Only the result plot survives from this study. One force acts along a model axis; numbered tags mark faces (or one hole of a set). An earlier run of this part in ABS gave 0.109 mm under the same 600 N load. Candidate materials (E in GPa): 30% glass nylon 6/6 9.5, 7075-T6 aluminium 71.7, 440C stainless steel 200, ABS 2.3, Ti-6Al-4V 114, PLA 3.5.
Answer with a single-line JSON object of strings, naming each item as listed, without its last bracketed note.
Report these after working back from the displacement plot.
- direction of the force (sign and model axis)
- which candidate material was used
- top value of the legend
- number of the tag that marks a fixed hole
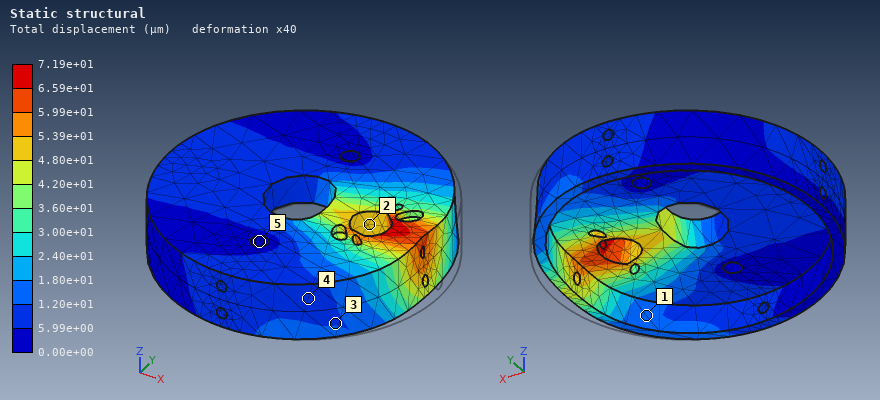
{"direction of the force": "-X", "which candidate material was used": "PLA", "top value of the legend": "7.19e+01 µm", "number of the tag that marks a fixed hole": "5"}
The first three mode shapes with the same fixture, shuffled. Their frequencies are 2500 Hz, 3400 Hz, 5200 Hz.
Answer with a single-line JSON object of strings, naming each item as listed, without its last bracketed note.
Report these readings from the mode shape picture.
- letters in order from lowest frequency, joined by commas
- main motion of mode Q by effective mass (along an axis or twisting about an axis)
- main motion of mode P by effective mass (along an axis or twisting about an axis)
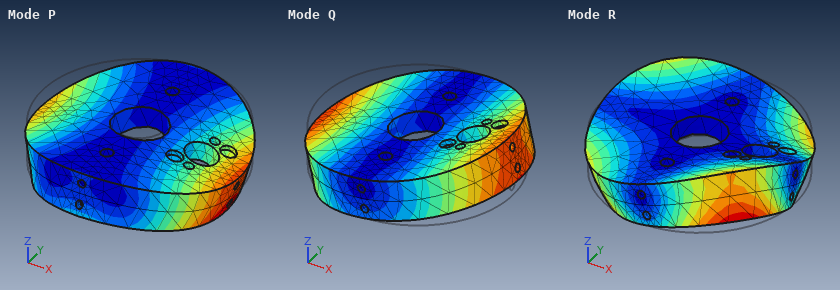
{"letters in order from lowest frequency, joined by commas": "Q, P, R", "main motion of mode Q by effective mass": "twisting about Y", "main motion of mode P by effective mass": "along Z"}
